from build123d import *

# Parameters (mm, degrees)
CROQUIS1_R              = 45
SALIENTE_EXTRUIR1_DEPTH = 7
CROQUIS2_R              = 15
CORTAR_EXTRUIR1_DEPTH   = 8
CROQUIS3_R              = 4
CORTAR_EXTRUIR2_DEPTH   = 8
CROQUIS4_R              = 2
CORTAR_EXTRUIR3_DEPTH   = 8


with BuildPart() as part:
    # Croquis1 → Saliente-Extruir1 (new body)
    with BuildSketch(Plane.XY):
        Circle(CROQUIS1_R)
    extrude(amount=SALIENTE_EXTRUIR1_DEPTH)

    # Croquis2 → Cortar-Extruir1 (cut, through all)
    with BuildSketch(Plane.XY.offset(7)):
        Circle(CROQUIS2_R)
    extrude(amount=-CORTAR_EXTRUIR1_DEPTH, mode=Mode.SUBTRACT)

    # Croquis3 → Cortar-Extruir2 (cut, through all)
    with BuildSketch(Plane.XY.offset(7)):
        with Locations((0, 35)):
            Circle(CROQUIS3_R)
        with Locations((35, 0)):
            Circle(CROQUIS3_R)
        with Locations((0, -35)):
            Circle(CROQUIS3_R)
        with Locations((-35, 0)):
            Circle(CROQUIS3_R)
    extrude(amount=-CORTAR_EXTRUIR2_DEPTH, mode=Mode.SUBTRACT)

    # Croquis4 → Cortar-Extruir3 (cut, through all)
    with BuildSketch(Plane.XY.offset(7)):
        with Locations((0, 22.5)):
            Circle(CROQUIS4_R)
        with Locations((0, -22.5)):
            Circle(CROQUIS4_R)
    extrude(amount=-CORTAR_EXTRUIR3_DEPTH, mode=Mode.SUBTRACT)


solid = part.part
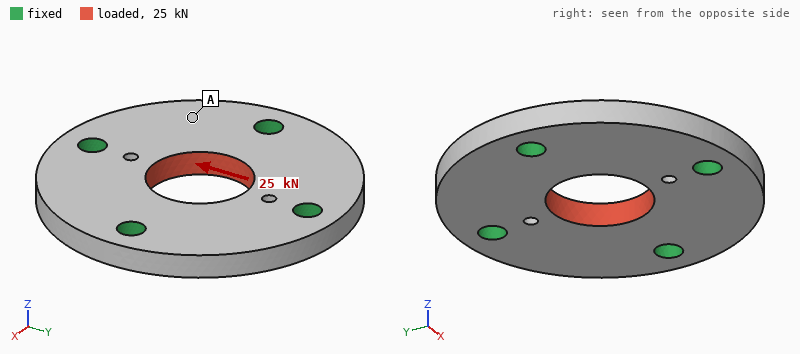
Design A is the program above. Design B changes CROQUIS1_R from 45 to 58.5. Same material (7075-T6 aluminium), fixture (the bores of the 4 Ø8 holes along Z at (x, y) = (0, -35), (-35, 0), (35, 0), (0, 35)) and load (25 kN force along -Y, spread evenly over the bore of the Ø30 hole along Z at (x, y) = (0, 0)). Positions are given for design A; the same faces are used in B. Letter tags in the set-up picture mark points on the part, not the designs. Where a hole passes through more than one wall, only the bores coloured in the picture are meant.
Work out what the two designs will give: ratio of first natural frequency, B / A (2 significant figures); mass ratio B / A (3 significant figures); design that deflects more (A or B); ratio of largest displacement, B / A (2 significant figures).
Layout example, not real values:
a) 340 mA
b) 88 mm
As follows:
a) 0.49
b) 1.81
c) A
d) 0.89
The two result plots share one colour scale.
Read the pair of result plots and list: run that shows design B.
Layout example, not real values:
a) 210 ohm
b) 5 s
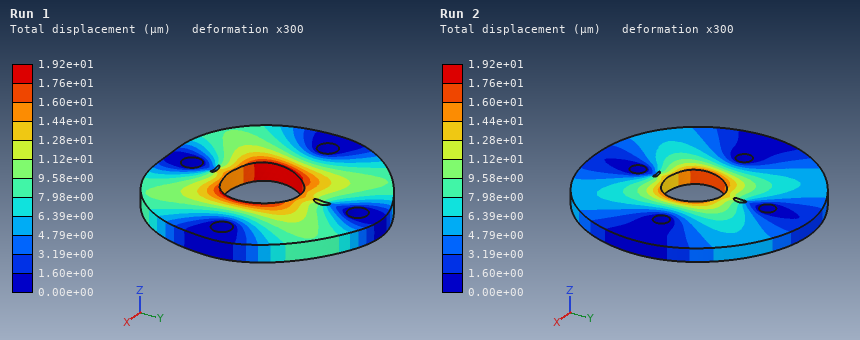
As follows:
a) Run 2
